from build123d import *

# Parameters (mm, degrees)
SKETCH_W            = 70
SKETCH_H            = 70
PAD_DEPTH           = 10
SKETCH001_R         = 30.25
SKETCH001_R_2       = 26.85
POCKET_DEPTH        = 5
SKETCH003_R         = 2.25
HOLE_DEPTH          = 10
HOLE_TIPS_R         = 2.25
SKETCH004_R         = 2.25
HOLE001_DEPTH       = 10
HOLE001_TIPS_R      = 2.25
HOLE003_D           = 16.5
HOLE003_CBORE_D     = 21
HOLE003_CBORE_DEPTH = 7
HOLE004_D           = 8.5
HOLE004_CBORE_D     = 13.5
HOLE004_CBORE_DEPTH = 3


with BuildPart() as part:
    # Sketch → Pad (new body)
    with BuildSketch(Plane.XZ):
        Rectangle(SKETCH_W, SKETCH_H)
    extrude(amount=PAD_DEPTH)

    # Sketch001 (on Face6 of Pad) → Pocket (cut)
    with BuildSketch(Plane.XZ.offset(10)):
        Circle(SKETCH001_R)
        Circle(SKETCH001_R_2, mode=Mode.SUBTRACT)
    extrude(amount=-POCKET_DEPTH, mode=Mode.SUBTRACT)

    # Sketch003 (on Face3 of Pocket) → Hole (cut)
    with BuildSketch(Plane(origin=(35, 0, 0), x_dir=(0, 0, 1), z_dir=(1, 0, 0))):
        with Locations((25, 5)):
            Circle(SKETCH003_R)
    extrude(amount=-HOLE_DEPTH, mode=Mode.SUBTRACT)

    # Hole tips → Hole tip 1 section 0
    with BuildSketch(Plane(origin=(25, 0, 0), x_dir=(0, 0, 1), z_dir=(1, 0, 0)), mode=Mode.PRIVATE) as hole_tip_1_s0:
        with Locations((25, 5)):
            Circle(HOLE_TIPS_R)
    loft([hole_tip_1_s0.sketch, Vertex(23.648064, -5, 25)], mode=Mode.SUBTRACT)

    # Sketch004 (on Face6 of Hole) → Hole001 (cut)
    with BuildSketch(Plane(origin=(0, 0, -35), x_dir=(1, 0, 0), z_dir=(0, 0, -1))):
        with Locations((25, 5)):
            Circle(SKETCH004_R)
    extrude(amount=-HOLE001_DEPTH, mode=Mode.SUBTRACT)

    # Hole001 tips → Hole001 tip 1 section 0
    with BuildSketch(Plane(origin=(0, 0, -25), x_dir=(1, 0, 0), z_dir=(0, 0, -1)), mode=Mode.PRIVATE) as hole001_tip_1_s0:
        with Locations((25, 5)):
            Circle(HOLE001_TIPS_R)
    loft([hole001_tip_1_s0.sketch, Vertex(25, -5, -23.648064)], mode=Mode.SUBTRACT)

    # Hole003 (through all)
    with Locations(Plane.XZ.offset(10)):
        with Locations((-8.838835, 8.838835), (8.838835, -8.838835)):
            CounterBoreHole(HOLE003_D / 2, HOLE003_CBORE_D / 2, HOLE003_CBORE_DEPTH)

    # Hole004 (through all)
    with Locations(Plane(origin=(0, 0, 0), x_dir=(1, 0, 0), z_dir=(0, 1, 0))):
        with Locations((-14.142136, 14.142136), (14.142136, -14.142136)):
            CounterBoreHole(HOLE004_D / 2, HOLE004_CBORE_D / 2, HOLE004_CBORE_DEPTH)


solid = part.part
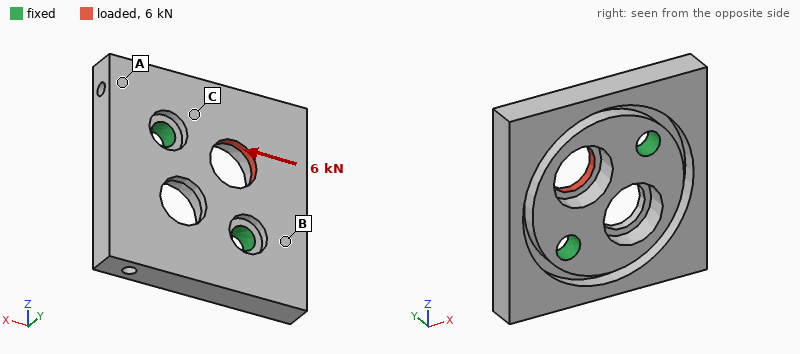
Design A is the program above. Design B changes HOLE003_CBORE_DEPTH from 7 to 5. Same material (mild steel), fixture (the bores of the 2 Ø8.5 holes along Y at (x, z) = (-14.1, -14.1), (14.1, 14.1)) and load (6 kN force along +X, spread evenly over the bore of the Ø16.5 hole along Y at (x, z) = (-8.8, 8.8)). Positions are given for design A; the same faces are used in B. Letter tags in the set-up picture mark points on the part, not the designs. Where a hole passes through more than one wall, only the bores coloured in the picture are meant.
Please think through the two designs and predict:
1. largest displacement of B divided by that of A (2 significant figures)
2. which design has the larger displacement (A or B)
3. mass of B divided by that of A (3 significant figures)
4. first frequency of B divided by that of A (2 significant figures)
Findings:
0.74
A
1.01
1.00
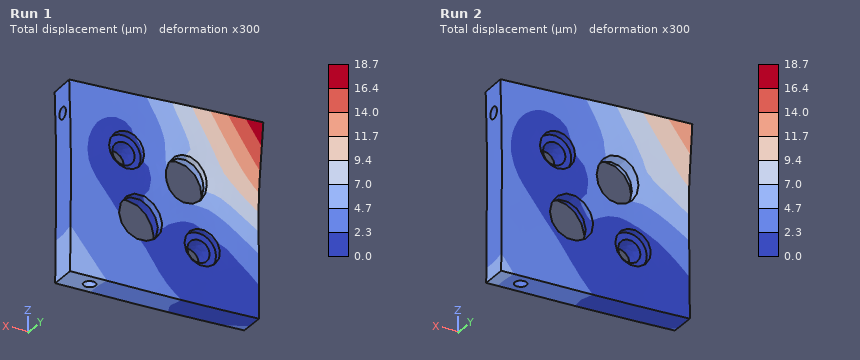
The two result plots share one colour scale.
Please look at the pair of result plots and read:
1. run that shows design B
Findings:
Run 2
